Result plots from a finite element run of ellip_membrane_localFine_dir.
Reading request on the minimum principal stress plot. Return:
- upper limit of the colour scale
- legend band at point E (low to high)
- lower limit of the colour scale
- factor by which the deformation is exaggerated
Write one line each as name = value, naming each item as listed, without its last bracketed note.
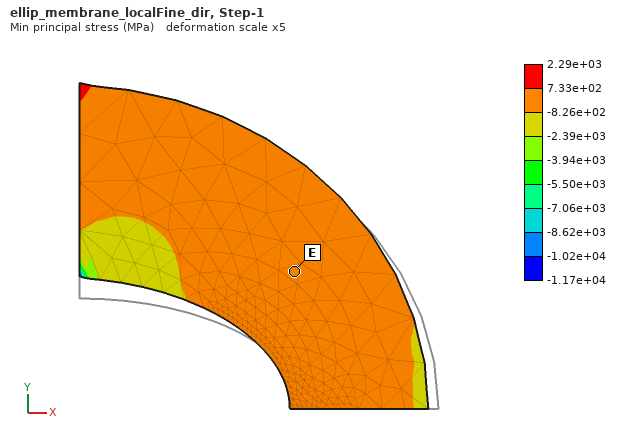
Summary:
upper limit of the colour scale = 2.29e+03 MPa
legend band at point E = -8.26e+02 to 7.33e+02 MPa
lower limit of the colour scale = -1.17e+04 MPa
factor by which the deformation is exaggerated = 5
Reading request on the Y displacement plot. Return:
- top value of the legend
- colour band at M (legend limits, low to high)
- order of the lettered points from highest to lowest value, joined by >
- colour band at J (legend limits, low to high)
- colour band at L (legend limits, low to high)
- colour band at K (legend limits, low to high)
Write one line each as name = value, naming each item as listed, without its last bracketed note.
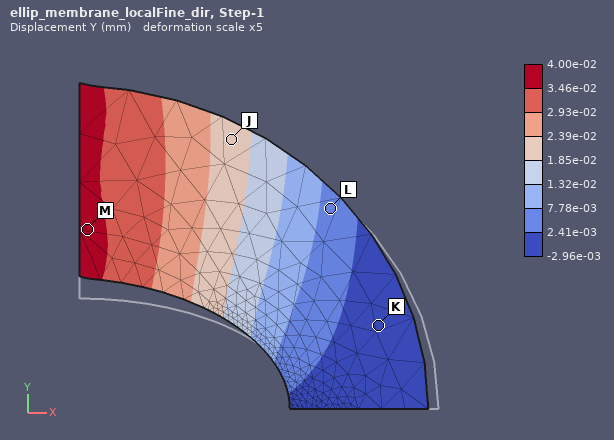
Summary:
top value of the legend = 4.00e-02 mm
colour band at M = 3.46e-02 to 4.00e-02 mm
order of the lettered points from highest to lowest value, joined by > = M > J > L > K
colour band at J = 1.85e-02 to 2.39e-02 mm
colour band at L = 2.41e-03 to 7.78e-03 mm
colour band at K = -2.96e-03 to 2.41e-03 mm
